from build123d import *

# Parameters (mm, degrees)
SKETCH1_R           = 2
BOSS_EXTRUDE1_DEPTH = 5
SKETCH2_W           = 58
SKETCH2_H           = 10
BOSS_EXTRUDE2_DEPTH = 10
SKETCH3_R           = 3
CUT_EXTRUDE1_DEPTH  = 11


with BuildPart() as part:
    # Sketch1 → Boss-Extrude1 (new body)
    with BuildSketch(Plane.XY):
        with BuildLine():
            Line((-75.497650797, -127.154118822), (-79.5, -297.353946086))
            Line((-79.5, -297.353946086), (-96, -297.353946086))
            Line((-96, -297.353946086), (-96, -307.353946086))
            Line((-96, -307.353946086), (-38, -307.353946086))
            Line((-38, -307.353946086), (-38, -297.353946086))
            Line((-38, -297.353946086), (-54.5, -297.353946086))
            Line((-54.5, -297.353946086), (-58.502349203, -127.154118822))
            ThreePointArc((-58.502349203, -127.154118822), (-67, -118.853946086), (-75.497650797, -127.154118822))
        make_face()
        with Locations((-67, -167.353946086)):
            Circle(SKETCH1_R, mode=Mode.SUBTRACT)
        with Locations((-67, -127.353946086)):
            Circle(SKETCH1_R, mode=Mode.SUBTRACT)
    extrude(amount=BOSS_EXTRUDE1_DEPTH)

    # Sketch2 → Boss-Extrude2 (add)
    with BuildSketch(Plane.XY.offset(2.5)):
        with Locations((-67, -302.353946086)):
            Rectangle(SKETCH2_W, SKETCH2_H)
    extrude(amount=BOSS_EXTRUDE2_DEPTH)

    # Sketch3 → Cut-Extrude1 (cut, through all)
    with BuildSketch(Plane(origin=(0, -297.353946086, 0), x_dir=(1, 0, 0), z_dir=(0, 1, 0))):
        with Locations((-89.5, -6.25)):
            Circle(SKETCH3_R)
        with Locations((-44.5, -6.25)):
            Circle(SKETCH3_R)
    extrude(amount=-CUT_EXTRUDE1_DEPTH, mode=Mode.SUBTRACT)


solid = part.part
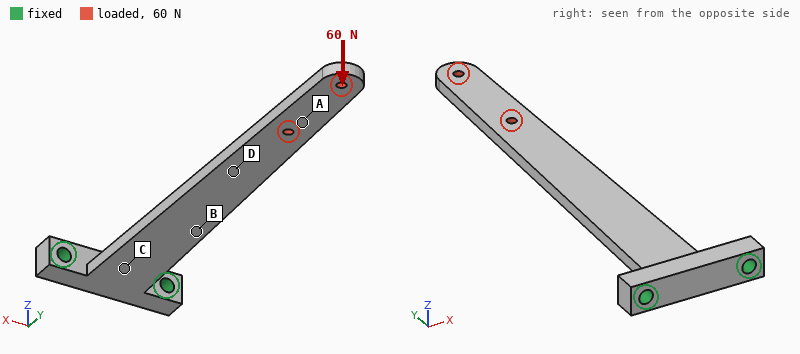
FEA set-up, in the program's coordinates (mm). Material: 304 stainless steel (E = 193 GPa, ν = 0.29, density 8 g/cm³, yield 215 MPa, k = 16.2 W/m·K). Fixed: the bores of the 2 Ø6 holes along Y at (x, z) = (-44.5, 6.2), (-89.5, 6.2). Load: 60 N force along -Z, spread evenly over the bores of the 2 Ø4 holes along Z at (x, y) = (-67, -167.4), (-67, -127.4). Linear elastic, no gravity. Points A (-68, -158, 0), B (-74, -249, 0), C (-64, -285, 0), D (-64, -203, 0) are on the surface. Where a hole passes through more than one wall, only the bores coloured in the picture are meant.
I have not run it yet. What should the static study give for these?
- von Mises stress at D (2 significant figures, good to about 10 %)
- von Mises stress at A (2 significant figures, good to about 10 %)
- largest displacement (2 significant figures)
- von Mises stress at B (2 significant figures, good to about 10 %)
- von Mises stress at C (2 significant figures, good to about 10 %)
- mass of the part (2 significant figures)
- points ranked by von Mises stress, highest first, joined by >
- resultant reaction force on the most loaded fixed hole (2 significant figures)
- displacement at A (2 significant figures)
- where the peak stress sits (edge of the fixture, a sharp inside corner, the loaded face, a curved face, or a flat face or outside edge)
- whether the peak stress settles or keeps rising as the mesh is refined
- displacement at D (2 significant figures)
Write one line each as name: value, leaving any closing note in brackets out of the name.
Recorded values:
von Mises stress at D: 39 MPa
von Mises stress at A: 12 MPa
largest displacement: 2.0 mm
von Mises stress at B: 64 MPa
von Mises stress at C: 78 MPa
mass of the part: 200 g
points ranked by von Mises stress, highest first, joined by >: C > B > D > A
resultant reaction force on the most loaded fixed hole: 36 N
displacement at A: 1.4 mm
where the peak stress sits: a sharp inside corner
whether the peak stress settles or keeps rising as the mesh is refined: keeps rising
displacement at D: 0.73 mm
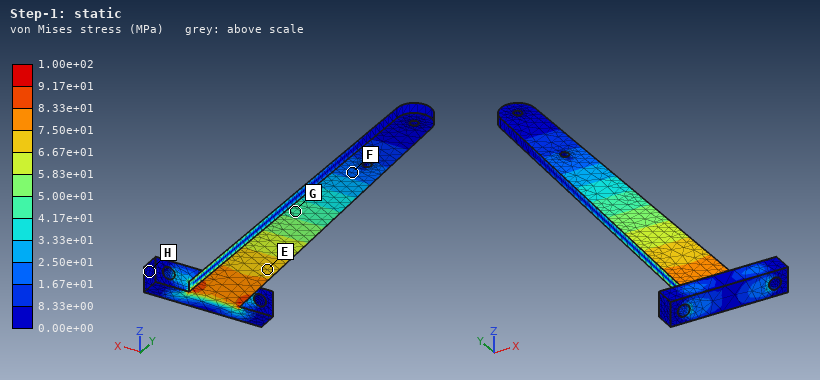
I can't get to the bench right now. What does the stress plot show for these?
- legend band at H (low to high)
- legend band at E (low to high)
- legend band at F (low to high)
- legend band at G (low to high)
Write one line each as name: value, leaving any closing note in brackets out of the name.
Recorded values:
legend band at H: 0.00e+00 to 8.33e+00 MPa
legend band at E: 6.67e+01 to 7.50e+01 MPa
legend band at F: 1.67e+01 to 2.50e+01 MPa
legend band at G: 4.17e+01 to 5.00e+01 MPa
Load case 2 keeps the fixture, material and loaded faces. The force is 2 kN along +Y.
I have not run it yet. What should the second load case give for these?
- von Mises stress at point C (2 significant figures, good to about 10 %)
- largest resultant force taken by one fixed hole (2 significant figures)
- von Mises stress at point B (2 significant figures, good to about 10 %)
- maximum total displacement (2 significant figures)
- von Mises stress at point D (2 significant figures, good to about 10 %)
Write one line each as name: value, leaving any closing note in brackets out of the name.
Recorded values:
von Mises stress at point C: 15 MPa
largest resultant force taken by one fixed hole: 1.0 kN
von Mises stress at point B: 18 MPa
maximum total displacement: 58 µm
von Mises stress at point D: 19 MPa
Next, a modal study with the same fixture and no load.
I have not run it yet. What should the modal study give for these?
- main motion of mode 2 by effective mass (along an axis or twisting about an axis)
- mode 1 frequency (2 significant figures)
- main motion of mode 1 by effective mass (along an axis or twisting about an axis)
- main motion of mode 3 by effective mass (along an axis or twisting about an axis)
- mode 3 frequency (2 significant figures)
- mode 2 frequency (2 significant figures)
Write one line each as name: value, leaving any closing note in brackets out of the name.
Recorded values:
main motion of mode 2 by effective mass: along X
mode 1 frequency: 140 Hz
main motion of mode 1 by effective mass: along Z
main motion of mode 3 by effective mass: along Z
mode 3 frequency: 790 Hz
mode 2 frequency: 610 Hz
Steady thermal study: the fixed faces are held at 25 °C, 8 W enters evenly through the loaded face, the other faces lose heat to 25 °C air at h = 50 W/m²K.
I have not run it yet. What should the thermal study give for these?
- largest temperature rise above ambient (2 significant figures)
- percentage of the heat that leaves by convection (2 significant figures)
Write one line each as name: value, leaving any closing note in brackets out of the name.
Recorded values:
largest temperature rise above ambient: 72 K
percentage of the heat that leaves by convection: 100 %
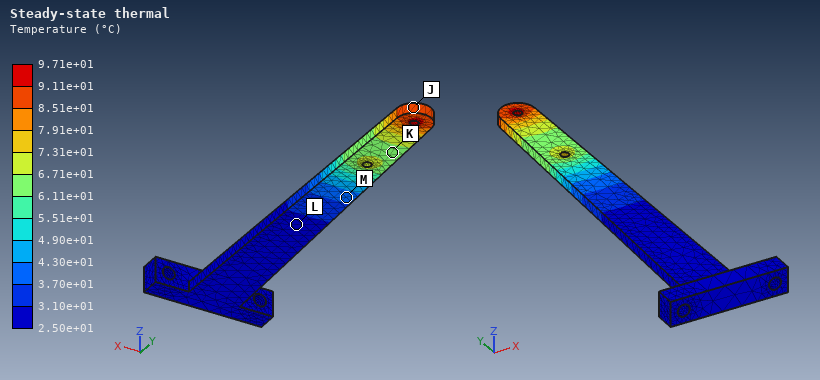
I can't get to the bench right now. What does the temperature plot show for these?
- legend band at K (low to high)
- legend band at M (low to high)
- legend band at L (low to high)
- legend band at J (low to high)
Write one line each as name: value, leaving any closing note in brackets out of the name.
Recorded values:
legend band at K: 6.11e+01 to 6.71e+01 °C
legend band at M: 3.70e+01 to 4.30e+01 °C
legend band at L: 2.50e+01 to 3.10e+01 °C
legend band at J: 8.51e+01 to 9.11e+01 °C
